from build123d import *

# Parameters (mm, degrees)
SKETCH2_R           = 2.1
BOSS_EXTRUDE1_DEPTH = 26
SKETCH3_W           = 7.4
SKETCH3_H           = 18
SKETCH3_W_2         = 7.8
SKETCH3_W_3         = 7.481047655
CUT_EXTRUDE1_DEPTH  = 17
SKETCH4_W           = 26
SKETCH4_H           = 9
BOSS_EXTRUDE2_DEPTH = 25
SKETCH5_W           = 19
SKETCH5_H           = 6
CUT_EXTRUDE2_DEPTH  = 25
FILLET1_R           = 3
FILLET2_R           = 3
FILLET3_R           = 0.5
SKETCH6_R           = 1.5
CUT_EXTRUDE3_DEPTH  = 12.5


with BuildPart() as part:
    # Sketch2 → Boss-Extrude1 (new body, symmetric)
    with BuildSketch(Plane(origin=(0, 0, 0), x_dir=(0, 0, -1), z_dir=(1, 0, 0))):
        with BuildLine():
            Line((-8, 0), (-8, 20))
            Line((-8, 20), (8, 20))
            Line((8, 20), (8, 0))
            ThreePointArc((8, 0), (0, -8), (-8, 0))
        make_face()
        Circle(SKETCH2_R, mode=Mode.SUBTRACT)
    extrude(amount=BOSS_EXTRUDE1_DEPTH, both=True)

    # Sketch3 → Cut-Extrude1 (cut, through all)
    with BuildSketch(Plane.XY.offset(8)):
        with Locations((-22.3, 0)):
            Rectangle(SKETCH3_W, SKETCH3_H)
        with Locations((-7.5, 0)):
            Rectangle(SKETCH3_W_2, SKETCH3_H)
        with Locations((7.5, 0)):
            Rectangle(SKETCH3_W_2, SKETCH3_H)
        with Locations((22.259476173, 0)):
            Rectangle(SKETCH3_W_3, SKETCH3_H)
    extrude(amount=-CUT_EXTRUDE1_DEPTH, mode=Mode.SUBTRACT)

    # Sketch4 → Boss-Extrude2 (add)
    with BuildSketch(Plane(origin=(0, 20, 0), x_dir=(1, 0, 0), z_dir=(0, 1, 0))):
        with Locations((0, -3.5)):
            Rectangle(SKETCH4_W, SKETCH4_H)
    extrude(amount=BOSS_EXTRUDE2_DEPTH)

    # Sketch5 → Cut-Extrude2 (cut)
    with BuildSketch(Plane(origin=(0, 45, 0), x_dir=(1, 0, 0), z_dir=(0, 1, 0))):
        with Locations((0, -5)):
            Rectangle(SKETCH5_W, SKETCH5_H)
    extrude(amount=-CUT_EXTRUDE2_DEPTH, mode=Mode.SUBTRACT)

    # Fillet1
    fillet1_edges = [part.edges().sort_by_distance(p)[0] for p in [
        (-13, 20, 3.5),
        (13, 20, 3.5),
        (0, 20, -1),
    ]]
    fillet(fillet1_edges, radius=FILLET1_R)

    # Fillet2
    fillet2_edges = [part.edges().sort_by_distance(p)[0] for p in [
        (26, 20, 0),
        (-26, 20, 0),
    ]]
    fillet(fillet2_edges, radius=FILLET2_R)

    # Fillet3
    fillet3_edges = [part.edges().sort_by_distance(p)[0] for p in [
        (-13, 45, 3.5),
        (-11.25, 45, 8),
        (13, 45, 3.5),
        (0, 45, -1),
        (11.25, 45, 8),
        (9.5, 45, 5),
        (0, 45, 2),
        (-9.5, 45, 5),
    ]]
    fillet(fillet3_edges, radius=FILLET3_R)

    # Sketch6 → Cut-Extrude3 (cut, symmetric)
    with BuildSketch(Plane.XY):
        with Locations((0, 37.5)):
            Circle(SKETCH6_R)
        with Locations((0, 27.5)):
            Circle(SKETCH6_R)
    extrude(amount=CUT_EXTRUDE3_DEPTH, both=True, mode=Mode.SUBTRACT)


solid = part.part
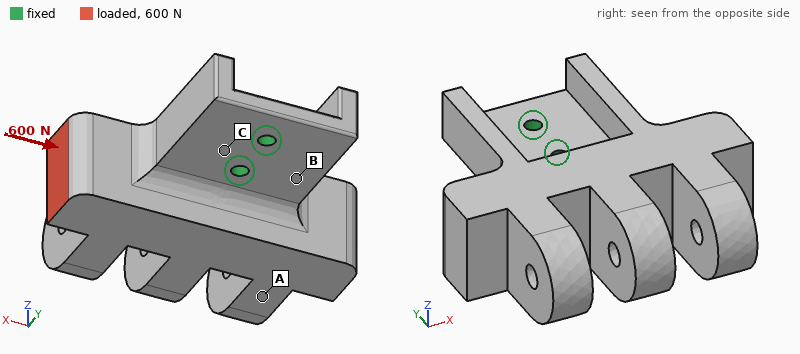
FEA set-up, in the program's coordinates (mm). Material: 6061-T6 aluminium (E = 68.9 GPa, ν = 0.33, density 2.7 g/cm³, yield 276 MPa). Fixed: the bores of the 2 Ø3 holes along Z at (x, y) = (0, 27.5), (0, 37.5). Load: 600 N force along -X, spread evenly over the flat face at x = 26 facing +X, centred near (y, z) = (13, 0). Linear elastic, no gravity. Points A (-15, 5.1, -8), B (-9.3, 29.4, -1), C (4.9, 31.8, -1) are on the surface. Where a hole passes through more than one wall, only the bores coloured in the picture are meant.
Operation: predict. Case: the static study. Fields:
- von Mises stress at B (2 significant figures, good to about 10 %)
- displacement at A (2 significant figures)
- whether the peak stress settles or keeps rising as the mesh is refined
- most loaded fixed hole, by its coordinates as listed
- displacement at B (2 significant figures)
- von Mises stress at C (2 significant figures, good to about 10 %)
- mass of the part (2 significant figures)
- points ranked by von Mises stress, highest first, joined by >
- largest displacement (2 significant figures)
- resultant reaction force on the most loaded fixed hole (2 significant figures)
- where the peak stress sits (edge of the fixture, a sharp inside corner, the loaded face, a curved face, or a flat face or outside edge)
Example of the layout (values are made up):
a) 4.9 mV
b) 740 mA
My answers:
a) 13 MPa
b) 25 µm
c) keeps rising
d) (0, 27.5)
e) 5.6 µm
f) 17 MPa
g) 46 g
h) C > B > A
i) 36 µm
j) 1.2 kN
k) edge of the fixture
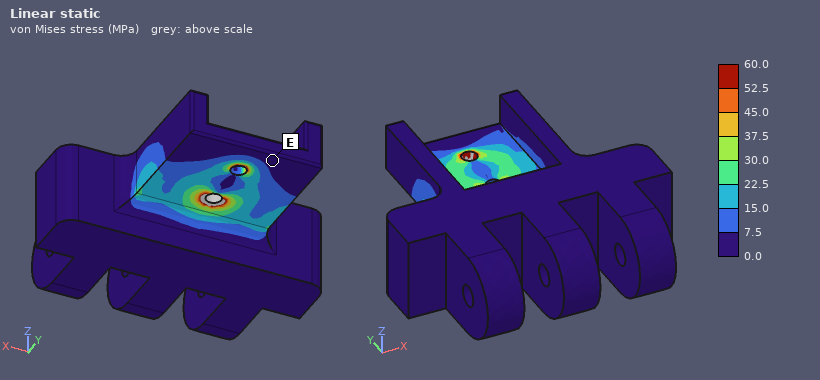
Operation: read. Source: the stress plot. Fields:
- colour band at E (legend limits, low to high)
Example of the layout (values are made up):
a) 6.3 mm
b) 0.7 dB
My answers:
a) 0.0 to 7.5 MPa
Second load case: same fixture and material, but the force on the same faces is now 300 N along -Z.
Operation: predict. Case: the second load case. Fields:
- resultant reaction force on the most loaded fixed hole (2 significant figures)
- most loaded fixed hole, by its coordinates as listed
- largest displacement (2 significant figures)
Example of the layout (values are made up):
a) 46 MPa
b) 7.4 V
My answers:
a) 530 N
b) (0, 27.5)
c) 0.20 mm
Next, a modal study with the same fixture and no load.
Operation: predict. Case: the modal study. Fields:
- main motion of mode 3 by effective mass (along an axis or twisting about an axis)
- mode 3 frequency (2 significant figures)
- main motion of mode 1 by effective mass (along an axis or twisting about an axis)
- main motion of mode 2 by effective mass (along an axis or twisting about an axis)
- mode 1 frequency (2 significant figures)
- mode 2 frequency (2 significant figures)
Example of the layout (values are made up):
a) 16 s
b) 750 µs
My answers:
a) along X
b) 3500 Hz
c) along Z
d) twisting about Y
e) 1900 Hz
f) 2000 Hz
